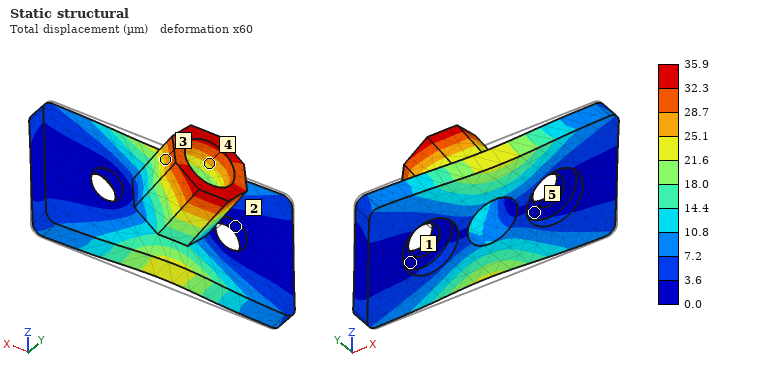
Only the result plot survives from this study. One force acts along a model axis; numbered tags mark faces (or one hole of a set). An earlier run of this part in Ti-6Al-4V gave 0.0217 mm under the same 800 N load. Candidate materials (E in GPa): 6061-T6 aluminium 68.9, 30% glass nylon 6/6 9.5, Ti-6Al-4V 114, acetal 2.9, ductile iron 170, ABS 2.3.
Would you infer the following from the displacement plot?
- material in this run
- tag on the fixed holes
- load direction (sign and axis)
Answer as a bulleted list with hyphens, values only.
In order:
- 6061-T6 aluminium
- 2
- +Z
